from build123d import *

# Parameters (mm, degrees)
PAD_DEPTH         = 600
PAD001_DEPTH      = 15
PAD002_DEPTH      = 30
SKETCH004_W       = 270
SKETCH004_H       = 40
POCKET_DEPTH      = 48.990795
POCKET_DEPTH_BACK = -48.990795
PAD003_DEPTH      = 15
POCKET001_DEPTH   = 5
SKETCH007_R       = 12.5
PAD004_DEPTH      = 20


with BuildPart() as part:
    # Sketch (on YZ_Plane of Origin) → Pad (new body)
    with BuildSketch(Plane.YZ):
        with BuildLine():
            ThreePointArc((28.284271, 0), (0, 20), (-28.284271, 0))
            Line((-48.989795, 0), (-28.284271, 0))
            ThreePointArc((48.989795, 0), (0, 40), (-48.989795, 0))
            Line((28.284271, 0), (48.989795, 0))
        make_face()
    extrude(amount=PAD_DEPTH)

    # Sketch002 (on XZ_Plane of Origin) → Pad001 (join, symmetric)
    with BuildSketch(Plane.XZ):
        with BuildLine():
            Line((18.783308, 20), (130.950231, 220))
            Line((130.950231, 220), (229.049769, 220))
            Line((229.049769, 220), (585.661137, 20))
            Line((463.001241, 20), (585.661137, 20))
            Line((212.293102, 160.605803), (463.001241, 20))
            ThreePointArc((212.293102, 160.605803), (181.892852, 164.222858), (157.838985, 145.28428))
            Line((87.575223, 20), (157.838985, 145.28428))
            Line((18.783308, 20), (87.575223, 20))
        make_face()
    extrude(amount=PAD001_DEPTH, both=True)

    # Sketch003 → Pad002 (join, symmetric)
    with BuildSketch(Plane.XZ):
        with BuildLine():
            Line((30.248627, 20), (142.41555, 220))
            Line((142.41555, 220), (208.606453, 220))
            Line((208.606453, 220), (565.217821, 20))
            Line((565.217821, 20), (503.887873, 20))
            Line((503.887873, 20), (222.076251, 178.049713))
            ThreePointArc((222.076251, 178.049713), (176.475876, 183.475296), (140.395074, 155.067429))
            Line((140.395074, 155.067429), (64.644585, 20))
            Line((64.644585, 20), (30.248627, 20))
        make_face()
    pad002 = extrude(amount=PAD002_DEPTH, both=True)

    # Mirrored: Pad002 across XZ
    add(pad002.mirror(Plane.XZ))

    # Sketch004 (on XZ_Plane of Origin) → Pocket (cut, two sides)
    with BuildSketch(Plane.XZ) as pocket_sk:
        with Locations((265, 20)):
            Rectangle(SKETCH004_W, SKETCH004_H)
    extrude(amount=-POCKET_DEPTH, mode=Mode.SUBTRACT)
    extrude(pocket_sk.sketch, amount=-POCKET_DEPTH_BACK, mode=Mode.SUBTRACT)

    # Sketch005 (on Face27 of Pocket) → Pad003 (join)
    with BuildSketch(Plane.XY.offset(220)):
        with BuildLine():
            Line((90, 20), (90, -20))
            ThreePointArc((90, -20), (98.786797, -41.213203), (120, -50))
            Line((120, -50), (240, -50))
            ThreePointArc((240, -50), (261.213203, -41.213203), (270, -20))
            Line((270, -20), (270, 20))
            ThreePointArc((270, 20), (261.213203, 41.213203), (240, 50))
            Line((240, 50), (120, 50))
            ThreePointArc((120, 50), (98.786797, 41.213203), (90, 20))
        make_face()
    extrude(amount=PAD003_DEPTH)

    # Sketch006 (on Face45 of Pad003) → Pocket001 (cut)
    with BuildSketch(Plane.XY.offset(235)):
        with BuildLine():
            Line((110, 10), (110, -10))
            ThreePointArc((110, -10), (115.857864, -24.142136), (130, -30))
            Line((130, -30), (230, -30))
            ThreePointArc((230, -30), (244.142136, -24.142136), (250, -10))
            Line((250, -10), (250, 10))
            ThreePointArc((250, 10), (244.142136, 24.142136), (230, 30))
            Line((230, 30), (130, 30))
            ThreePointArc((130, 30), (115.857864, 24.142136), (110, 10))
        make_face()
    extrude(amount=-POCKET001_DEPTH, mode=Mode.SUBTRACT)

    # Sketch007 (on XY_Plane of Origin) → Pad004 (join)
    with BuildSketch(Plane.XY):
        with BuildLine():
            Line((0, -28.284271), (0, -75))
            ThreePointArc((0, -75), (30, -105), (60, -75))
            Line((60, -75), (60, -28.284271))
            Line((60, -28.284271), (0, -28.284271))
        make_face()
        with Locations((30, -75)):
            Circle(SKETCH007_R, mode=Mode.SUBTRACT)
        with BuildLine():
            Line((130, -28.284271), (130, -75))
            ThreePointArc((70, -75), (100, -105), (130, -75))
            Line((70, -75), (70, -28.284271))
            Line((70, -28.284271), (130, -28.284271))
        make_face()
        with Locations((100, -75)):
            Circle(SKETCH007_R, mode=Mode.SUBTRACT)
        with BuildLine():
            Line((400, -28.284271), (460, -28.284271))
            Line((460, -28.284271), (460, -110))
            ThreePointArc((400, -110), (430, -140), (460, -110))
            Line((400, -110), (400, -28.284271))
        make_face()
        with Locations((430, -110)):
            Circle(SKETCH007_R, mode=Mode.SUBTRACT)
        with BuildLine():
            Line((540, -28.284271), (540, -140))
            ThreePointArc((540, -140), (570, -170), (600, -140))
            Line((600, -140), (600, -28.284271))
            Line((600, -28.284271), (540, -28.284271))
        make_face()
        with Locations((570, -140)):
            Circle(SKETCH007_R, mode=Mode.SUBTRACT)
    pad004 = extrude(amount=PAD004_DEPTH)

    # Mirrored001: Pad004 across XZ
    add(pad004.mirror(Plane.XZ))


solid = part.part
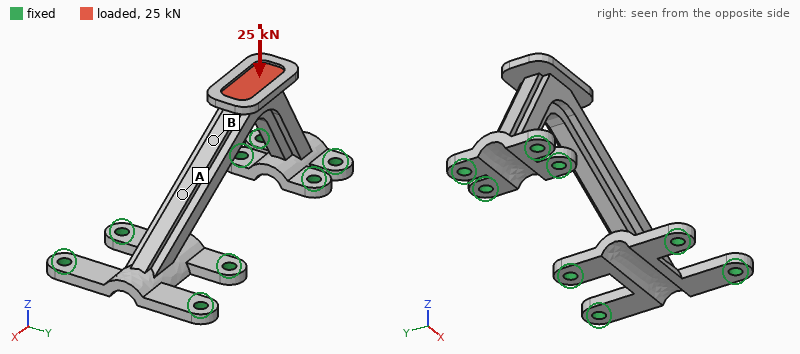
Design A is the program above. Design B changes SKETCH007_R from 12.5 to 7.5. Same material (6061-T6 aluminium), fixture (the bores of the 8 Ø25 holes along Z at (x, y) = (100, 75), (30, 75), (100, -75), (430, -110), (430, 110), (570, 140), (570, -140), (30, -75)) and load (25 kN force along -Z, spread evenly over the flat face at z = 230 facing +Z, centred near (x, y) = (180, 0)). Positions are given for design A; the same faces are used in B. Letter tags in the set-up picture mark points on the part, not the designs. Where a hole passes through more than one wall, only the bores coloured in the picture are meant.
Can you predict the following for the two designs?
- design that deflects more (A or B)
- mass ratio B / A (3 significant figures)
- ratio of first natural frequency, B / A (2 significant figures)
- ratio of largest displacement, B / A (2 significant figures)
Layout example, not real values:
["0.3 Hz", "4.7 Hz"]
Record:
["B", "1.02", "0.98", "1.1"]
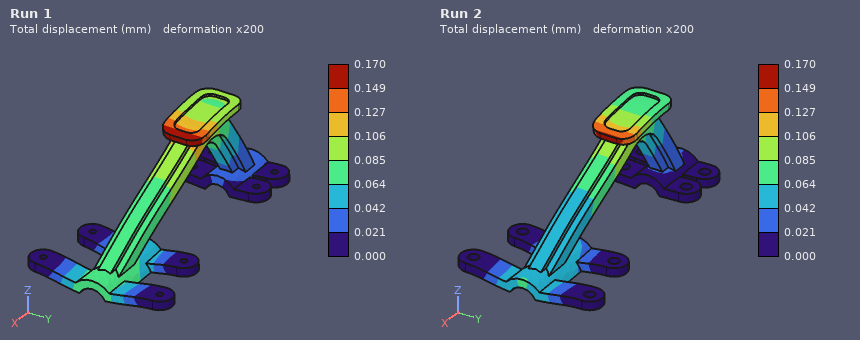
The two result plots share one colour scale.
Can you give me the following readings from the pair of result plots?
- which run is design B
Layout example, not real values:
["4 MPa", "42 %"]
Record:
["Run 1"]
